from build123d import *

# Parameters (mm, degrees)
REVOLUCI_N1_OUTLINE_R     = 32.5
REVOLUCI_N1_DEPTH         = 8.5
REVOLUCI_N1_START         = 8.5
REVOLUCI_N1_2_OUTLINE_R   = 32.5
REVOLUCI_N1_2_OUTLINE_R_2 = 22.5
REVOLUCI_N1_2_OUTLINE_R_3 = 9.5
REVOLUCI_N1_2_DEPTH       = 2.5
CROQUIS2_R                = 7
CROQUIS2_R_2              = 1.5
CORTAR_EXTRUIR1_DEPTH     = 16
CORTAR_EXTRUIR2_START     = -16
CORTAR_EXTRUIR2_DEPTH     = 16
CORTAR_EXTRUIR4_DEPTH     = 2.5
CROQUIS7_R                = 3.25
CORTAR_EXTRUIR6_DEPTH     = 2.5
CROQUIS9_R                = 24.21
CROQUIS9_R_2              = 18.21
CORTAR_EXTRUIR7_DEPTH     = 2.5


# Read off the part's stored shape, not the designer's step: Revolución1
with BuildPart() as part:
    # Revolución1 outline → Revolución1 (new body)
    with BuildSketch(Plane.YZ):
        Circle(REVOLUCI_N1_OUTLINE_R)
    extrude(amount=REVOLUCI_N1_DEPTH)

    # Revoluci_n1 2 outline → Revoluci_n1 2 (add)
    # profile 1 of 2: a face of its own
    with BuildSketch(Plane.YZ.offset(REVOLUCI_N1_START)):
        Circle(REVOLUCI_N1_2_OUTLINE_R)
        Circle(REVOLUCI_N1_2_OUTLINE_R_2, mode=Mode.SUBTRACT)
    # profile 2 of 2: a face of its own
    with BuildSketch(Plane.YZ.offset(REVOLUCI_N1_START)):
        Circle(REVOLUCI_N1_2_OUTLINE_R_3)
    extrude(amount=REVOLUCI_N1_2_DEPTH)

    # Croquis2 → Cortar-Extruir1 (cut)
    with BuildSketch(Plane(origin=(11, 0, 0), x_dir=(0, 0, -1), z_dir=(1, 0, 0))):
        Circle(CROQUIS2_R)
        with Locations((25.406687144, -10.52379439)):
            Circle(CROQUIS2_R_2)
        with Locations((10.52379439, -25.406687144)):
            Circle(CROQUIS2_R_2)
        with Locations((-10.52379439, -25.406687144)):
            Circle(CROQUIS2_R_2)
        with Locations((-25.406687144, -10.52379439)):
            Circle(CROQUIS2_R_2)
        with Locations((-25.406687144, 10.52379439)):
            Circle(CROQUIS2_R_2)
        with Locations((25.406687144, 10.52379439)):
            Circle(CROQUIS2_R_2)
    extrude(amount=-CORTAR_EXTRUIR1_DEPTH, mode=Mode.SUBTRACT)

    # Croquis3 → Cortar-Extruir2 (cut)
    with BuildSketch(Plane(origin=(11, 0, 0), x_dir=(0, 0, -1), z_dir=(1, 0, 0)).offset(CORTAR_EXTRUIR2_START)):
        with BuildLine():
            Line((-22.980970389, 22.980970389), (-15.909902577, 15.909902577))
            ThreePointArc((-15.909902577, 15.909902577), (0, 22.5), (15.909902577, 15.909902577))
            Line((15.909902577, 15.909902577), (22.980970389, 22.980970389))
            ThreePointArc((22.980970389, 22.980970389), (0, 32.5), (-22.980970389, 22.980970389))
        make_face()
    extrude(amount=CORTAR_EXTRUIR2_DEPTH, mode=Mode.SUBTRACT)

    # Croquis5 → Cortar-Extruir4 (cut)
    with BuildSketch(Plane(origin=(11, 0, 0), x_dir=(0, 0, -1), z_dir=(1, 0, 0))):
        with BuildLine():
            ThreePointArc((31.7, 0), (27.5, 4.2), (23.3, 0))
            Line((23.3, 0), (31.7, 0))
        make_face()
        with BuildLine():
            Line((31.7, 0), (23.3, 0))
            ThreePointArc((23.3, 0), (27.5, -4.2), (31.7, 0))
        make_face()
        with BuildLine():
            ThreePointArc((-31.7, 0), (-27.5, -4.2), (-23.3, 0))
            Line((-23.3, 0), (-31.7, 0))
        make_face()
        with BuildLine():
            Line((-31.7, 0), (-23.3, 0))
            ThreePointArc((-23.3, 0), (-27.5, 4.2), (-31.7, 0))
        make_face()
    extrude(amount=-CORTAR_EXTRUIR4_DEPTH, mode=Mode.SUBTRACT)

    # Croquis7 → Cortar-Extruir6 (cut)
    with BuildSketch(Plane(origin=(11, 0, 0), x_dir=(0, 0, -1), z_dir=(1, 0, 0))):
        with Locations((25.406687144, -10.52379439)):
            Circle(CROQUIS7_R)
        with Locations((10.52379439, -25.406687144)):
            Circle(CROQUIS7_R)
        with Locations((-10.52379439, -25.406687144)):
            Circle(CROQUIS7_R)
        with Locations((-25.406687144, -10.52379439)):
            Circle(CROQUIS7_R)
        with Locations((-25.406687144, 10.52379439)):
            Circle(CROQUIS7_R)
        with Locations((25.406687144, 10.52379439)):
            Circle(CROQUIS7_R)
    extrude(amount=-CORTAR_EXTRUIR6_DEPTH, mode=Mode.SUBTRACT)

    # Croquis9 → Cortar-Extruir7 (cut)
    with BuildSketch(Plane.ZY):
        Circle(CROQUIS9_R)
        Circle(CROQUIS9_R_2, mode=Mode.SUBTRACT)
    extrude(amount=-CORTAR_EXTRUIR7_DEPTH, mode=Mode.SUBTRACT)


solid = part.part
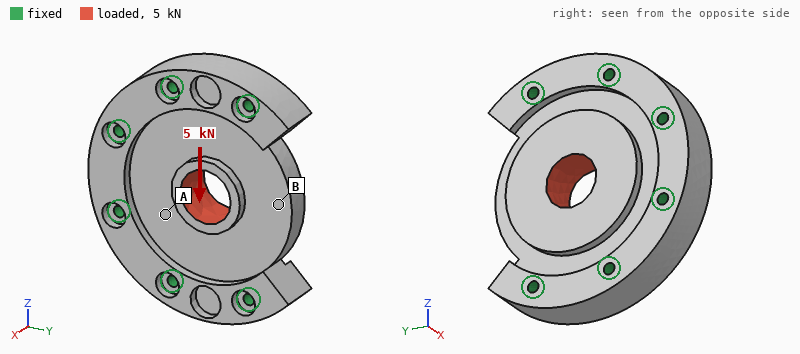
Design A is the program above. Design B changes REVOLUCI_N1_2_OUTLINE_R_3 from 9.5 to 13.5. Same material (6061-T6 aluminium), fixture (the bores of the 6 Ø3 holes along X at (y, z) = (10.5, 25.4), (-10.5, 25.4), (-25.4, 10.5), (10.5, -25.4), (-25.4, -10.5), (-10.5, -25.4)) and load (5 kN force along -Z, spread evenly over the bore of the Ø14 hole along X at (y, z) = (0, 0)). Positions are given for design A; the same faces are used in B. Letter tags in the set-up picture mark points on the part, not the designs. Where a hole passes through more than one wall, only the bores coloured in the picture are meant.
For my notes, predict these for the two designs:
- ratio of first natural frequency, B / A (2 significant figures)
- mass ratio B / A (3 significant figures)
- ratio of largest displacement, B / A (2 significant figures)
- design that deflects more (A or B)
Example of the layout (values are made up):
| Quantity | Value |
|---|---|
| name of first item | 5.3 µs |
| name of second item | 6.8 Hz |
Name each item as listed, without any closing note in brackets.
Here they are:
| Quantity | Value |
|---|---|
| ratio of first natural frequency, B / A | 1.0 |
| mass ratio B / A | 1.03 |
| ratio of largest displacement, B / A | 0.71 |
| design that deflects more | A |
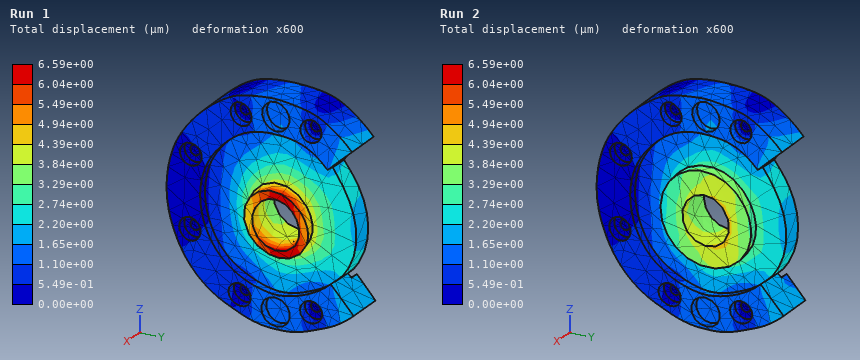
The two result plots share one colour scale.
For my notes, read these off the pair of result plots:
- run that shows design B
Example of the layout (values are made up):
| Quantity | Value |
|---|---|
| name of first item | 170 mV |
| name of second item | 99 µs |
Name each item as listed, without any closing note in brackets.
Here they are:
| Quantity | Value |
|---|---|
| run that shows design B | Run 2 |
